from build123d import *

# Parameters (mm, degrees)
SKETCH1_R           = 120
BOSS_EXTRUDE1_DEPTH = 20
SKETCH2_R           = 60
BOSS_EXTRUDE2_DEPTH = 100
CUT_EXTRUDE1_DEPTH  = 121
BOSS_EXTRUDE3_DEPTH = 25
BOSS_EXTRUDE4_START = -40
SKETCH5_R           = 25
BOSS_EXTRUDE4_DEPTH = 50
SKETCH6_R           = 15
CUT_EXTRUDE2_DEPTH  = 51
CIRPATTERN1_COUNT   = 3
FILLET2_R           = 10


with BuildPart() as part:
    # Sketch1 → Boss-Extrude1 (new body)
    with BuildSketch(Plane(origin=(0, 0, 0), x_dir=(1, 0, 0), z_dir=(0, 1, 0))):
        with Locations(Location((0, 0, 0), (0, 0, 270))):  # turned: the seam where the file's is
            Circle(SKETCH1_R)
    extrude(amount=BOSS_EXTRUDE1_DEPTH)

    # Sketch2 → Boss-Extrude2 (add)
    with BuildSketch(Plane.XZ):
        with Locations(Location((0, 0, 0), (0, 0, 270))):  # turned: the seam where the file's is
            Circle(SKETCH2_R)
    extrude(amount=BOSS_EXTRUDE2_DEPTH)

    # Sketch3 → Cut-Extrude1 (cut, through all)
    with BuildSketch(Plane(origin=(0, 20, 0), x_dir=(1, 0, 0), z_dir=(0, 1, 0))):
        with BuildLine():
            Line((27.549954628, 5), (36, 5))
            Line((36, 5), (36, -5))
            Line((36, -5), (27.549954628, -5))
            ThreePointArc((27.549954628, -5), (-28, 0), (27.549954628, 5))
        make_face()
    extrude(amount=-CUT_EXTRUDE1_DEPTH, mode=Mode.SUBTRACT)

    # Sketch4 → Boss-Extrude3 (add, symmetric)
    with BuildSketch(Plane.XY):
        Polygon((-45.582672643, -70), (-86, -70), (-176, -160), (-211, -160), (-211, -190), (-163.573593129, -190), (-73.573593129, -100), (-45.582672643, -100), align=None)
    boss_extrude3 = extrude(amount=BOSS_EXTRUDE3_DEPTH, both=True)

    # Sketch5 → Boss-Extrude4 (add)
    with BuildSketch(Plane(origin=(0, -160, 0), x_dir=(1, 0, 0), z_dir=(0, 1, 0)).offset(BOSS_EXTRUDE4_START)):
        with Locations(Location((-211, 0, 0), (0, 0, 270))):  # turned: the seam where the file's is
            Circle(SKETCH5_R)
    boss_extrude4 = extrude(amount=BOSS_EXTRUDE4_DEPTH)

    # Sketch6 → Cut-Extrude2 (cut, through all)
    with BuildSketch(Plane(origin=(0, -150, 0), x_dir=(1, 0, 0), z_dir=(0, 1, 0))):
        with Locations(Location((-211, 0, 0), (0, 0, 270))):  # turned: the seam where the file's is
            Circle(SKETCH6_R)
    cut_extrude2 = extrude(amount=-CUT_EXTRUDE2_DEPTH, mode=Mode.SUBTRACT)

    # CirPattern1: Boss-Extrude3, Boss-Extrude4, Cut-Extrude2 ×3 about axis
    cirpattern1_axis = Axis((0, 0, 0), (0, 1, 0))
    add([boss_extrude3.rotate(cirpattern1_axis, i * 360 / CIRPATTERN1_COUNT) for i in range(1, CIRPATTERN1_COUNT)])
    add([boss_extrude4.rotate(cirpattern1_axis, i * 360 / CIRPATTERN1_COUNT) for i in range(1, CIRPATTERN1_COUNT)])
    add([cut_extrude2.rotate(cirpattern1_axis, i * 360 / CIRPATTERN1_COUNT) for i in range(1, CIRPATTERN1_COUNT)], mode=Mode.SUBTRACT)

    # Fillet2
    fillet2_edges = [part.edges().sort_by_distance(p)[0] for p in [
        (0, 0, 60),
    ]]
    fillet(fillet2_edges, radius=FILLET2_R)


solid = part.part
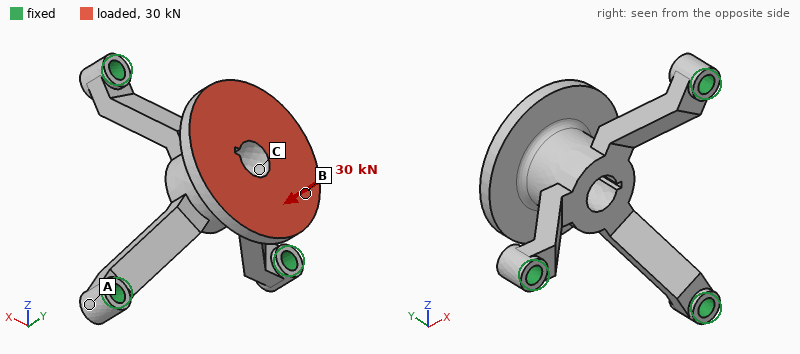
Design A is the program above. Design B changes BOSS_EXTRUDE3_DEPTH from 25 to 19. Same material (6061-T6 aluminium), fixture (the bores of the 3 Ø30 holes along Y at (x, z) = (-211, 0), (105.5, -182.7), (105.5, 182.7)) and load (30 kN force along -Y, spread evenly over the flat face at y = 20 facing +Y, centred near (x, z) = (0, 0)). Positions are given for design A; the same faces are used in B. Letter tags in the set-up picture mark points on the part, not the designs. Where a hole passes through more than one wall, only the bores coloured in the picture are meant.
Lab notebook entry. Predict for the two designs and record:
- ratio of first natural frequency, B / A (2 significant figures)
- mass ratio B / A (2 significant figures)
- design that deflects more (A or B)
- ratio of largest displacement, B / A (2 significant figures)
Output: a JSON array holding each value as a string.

["0.88", "0.93", "B", "1.1"]
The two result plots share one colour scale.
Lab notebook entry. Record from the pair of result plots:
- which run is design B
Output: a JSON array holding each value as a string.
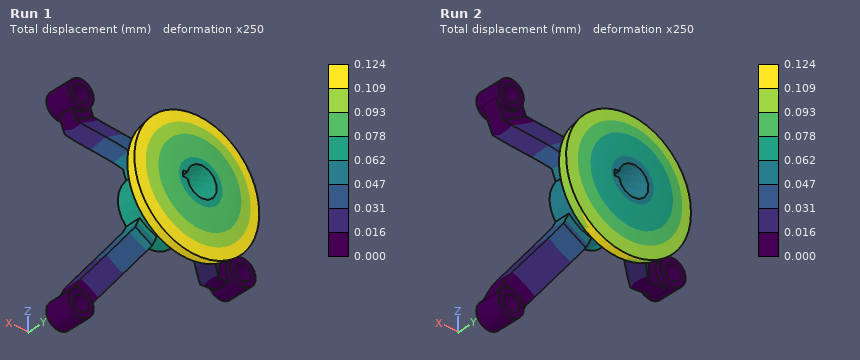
["Run 1"]
